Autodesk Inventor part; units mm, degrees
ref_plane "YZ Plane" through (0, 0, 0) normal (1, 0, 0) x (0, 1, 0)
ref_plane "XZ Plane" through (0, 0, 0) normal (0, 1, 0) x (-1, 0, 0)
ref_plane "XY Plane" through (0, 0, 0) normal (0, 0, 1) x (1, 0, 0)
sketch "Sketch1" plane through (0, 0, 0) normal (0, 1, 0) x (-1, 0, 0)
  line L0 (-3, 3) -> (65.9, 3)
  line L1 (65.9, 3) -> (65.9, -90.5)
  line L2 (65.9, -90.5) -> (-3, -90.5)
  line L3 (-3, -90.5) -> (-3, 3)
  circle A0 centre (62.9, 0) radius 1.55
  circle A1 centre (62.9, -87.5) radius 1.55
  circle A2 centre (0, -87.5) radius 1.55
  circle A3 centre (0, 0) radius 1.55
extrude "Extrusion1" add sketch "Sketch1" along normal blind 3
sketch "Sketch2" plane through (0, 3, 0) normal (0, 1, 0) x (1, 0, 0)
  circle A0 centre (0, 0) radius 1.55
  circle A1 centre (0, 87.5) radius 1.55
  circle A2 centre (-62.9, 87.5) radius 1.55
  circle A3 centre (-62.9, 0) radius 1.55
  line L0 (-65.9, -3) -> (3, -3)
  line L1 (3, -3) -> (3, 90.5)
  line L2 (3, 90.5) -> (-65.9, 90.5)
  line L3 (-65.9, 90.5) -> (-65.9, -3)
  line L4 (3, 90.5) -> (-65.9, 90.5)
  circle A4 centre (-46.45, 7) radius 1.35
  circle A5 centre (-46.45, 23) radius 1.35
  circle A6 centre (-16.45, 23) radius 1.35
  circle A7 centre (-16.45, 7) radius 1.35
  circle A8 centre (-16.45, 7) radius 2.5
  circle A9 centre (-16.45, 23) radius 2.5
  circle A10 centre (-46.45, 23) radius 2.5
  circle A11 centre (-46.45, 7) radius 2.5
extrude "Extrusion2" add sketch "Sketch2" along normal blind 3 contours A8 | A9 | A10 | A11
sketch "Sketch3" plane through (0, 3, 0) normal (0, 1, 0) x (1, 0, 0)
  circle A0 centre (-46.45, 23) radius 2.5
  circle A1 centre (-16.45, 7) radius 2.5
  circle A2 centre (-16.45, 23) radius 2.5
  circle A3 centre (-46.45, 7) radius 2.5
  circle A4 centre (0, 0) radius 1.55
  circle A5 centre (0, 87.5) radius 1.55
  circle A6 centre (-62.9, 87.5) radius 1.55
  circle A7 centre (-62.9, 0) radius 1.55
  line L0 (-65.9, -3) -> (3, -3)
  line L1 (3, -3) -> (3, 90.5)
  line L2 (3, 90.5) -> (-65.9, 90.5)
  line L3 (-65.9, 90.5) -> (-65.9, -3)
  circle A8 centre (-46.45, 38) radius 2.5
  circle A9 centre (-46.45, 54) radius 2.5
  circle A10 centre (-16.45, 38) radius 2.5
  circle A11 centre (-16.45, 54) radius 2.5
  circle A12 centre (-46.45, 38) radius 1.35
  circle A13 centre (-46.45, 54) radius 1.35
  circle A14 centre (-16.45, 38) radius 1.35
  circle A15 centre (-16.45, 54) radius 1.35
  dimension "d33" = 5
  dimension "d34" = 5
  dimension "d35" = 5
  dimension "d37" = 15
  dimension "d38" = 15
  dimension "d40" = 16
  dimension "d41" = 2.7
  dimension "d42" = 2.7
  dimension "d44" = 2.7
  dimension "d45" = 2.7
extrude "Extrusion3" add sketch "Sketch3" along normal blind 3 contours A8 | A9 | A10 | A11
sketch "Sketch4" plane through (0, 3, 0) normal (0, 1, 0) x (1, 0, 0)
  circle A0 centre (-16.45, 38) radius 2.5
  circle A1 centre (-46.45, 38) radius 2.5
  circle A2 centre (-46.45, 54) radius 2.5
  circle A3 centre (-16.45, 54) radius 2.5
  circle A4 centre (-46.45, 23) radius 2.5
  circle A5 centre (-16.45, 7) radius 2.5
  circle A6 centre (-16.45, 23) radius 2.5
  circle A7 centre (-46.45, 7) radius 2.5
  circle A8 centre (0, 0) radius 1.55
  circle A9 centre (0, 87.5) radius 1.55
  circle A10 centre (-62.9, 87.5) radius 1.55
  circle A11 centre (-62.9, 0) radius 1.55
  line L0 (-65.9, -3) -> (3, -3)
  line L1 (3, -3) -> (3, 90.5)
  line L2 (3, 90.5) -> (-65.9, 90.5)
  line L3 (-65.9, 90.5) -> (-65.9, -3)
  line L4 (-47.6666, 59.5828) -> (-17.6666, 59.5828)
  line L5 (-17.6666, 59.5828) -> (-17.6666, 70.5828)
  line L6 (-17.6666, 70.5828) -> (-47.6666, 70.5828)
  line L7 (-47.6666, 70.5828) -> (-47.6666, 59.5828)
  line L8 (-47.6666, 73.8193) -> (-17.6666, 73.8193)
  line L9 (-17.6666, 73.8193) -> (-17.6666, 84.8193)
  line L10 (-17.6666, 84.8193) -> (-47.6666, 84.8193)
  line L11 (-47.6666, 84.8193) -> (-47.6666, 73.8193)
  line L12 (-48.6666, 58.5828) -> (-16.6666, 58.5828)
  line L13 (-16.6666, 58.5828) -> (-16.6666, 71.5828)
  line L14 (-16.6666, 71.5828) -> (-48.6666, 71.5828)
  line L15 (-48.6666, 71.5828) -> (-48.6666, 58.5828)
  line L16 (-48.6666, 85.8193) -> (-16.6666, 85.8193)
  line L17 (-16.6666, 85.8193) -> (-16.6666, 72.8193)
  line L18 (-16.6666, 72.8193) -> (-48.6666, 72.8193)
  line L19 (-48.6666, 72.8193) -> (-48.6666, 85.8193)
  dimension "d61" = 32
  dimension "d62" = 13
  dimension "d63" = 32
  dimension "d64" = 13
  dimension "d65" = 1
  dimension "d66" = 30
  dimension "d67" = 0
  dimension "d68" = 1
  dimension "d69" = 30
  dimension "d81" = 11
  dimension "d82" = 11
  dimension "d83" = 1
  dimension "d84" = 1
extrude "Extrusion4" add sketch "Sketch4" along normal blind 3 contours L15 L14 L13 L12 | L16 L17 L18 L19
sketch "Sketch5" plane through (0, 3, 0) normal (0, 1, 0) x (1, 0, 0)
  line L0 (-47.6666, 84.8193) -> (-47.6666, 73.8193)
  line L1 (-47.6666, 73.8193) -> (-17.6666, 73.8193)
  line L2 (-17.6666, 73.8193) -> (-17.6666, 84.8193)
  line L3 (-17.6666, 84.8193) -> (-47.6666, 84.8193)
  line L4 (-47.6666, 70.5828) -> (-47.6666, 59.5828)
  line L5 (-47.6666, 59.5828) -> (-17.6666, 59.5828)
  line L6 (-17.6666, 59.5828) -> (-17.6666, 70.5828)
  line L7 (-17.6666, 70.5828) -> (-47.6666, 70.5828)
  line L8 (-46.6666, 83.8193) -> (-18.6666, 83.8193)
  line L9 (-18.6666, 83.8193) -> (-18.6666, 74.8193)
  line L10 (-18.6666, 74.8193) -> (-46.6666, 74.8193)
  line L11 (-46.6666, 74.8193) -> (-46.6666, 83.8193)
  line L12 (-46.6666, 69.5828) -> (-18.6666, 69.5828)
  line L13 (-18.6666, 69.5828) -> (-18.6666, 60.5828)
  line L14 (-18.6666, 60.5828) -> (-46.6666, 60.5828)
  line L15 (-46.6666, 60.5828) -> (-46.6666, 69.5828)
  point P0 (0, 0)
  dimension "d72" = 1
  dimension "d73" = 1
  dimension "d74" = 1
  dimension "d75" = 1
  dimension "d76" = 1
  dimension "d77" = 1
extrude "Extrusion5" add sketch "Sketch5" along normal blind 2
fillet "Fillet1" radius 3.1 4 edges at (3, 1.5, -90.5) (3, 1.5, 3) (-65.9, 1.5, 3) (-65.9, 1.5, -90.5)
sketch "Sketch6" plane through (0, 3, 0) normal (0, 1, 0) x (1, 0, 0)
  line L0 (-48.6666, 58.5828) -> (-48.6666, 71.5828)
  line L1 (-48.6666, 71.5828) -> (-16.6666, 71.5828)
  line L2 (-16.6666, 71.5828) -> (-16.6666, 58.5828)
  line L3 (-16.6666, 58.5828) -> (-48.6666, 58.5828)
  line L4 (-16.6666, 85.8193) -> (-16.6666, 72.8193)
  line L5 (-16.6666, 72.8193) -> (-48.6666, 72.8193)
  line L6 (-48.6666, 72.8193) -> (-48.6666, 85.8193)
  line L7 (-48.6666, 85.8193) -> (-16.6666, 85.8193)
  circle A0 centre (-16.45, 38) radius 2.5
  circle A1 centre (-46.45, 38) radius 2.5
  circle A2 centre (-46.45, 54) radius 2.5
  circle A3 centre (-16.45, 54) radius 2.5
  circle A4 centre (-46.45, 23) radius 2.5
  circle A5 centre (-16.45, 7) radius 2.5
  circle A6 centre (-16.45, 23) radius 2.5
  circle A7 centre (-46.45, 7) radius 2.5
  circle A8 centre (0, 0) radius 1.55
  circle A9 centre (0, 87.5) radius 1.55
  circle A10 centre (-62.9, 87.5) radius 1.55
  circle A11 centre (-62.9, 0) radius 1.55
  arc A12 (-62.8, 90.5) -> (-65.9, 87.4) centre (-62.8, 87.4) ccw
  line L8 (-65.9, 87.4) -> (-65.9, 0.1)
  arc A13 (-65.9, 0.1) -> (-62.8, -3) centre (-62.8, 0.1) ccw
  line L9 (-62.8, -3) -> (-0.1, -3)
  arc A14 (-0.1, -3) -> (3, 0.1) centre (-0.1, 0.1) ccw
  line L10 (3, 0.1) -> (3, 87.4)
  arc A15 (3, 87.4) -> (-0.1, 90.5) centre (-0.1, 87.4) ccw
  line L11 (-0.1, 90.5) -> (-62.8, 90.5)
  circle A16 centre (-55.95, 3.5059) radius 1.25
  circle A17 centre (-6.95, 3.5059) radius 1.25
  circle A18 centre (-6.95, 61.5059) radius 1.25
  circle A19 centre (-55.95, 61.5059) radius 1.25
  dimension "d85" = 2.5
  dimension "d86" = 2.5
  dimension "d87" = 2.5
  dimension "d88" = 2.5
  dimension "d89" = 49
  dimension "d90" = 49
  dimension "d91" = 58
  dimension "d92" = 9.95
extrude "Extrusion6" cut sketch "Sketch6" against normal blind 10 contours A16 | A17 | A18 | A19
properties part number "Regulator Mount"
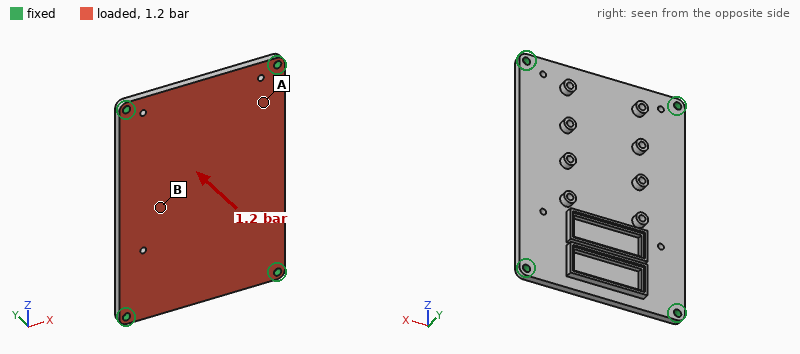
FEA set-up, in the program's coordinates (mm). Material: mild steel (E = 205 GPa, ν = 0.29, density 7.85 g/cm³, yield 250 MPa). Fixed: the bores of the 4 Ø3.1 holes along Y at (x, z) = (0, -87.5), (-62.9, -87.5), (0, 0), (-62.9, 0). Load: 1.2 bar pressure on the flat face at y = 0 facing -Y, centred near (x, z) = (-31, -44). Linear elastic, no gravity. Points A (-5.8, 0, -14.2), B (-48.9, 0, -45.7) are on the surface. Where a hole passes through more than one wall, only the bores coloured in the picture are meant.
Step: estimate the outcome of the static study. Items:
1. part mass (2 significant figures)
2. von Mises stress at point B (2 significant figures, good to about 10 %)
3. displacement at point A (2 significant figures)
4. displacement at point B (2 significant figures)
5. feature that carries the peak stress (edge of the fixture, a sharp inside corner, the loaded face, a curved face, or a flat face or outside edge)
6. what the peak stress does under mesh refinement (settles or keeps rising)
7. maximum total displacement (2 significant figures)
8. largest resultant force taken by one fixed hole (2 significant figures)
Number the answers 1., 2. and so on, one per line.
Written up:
1. 160 g
2. 32 MPa
3. 28 µm
4. 72 µm
5. edge of the fixture
6. keeps rising
7. 76 µm
8. 200 N
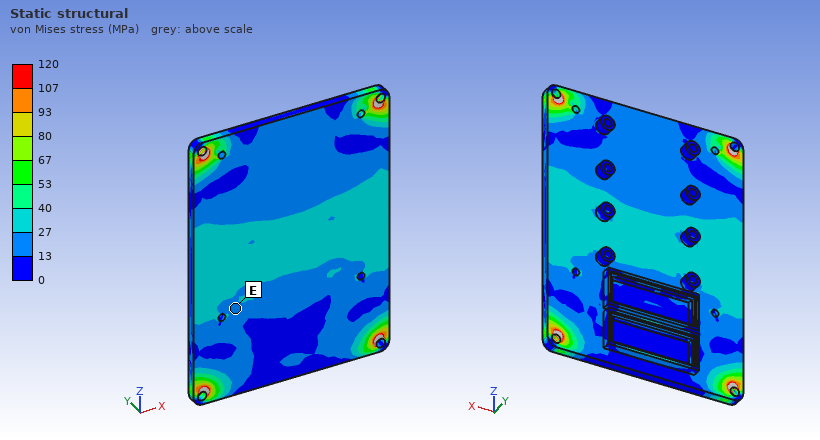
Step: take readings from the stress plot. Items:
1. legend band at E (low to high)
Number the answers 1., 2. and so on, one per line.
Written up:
1. 13 to 27 MPa
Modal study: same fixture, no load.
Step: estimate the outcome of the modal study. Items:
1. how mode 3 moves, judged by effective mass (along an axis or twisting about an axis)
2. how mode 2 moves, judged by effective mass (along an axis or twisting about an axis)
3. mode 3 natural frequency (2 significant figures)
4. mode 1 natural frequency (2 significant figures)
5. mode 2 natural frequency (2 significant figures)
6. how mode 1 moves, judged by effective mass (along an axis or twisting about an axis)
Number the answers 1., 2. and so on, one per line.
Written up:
1. twisting about X
2. twisting about Z
3. 3500 Hz
4. 1500 Hz
5. 2600 Hz
6. along Y
